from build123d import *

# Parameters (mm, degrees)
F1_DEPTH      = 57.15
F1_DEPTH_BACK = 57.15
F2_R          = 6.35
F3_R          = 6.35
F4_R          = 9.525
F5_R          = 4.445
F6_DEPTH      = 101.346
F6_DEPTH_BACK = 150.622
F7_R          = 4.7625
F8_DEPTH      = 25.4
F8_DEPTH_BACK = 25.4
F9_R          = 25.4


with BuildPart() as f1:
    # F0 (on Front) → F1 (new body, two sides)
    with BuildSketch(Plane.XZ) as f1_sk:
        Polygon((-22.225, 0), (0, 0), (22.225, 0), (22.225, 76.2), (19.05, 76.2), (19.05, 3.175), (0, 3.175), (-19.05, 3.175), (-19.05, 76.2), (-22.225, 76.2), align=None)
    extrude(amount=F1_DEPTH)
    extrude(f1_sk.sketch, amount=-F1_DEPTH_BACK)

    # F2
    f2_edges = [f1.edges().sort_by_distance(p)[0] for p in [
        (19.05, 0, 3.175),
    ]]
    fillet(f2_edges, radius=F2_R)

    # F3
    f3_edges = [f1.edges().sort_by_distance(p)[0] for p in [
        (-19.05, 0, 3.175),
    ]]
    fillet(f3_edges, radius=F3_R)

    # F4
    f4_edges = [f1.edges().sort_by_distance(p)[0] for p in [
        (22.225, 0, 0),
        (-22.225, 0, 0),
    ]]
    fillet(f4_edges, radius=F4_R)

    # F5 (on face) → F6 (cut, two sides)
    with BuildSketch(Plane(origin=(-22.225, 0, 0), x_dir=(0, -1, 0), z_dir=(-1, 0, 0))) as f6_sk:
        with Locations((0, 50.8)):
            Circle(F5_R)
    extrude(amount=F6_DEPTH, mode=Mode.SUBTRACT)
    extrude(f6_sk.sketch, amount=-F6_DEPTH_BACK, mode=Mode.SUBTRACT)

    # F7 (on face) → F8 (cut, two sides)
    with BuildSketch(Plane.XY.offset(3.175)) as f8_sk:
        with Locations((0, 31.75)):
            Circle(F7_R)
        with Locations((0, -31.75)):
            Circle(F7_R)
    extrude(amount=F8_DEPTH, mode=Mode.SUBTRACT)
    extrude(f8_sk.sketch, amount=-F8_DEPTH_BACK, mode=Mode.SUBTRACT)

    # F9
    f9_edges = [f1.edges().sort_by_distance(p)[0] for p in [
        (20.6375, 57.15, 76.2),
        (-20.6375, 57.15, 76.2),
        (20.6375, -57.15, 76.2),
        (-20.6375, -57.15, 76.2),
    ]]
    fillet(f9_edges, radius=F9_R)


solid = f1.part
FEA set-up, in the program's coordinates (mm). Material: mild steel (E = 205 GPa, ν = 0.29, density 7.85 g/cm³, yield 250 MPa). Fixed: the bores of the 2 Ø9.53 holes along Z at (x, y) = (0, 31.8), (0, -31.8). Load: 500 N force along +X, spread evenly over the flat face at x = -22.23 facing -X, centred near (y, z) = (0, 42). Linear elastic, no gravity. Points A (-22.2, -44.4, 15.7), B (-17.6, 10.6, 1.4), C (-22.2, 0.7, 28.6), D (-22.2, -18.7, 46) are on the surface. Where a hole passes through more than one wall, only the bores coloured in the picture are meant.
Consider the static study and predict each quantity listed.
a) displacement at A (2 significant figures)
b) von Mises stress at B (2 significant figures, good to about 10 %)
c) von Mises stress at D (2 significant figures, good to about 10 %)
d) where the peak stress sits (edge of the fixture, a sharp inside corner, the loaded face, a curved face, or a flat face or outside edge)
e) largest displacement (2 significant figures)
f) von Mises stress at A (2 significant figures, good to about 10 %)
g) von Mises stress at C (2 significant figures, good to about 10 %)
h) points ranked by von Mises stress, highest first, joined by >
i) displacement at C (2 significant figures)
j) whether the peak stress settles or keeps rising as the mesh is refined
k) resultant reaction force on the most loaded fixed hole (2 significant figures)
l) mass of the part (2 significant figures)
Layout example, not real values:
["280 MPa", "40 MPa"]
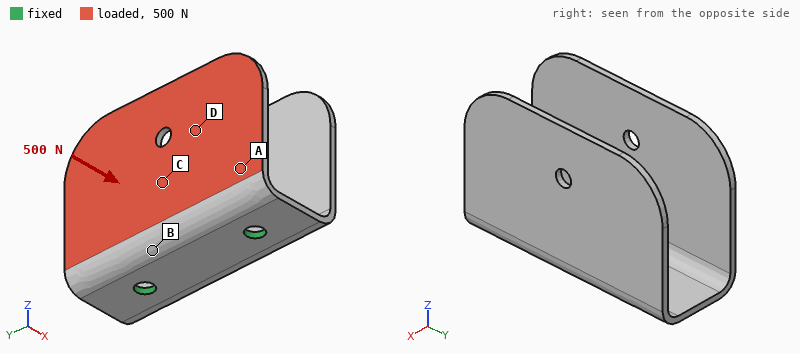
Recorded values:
["0.12 mm", "82 MPa", "16 MPa", "edge of the fixture", "0.80 mm", "60 MPa", "37 MPa", "B > A > C > D", "0.23 mm", "keeps rising", "250 N", "500 g"]
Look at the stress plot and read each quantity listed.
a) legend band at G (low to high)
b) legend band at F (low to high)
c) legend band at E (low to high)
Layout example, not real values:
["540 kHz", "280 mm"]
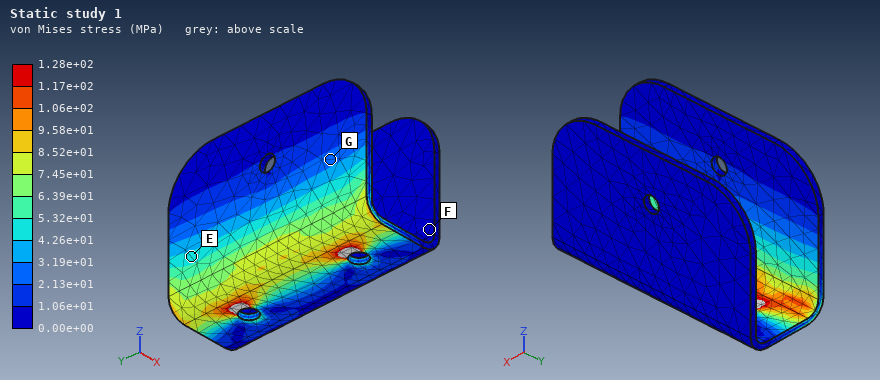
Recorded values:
["2.13e+01 to 3.19e+01 MPa", "0.00e+00 to 1.06e+01 MPa", "4.26e+01 to 5.32e+01 MPa"]
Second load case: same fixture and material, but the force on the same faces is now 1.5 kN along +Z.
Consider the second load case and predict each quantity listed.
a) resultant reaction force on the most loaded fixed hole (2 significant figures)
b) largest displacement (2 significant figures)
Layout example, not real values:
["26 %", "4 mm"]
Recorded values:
["750 N", "0.47 mm"]
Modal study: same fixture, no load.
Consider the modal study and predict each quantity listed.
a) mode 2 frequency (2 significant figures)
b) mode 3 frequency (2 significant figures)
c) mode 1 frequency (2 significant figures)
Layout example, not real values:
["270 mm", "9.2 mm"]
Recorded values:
["380 Hz", "770 Hz", "360 Hz"]
